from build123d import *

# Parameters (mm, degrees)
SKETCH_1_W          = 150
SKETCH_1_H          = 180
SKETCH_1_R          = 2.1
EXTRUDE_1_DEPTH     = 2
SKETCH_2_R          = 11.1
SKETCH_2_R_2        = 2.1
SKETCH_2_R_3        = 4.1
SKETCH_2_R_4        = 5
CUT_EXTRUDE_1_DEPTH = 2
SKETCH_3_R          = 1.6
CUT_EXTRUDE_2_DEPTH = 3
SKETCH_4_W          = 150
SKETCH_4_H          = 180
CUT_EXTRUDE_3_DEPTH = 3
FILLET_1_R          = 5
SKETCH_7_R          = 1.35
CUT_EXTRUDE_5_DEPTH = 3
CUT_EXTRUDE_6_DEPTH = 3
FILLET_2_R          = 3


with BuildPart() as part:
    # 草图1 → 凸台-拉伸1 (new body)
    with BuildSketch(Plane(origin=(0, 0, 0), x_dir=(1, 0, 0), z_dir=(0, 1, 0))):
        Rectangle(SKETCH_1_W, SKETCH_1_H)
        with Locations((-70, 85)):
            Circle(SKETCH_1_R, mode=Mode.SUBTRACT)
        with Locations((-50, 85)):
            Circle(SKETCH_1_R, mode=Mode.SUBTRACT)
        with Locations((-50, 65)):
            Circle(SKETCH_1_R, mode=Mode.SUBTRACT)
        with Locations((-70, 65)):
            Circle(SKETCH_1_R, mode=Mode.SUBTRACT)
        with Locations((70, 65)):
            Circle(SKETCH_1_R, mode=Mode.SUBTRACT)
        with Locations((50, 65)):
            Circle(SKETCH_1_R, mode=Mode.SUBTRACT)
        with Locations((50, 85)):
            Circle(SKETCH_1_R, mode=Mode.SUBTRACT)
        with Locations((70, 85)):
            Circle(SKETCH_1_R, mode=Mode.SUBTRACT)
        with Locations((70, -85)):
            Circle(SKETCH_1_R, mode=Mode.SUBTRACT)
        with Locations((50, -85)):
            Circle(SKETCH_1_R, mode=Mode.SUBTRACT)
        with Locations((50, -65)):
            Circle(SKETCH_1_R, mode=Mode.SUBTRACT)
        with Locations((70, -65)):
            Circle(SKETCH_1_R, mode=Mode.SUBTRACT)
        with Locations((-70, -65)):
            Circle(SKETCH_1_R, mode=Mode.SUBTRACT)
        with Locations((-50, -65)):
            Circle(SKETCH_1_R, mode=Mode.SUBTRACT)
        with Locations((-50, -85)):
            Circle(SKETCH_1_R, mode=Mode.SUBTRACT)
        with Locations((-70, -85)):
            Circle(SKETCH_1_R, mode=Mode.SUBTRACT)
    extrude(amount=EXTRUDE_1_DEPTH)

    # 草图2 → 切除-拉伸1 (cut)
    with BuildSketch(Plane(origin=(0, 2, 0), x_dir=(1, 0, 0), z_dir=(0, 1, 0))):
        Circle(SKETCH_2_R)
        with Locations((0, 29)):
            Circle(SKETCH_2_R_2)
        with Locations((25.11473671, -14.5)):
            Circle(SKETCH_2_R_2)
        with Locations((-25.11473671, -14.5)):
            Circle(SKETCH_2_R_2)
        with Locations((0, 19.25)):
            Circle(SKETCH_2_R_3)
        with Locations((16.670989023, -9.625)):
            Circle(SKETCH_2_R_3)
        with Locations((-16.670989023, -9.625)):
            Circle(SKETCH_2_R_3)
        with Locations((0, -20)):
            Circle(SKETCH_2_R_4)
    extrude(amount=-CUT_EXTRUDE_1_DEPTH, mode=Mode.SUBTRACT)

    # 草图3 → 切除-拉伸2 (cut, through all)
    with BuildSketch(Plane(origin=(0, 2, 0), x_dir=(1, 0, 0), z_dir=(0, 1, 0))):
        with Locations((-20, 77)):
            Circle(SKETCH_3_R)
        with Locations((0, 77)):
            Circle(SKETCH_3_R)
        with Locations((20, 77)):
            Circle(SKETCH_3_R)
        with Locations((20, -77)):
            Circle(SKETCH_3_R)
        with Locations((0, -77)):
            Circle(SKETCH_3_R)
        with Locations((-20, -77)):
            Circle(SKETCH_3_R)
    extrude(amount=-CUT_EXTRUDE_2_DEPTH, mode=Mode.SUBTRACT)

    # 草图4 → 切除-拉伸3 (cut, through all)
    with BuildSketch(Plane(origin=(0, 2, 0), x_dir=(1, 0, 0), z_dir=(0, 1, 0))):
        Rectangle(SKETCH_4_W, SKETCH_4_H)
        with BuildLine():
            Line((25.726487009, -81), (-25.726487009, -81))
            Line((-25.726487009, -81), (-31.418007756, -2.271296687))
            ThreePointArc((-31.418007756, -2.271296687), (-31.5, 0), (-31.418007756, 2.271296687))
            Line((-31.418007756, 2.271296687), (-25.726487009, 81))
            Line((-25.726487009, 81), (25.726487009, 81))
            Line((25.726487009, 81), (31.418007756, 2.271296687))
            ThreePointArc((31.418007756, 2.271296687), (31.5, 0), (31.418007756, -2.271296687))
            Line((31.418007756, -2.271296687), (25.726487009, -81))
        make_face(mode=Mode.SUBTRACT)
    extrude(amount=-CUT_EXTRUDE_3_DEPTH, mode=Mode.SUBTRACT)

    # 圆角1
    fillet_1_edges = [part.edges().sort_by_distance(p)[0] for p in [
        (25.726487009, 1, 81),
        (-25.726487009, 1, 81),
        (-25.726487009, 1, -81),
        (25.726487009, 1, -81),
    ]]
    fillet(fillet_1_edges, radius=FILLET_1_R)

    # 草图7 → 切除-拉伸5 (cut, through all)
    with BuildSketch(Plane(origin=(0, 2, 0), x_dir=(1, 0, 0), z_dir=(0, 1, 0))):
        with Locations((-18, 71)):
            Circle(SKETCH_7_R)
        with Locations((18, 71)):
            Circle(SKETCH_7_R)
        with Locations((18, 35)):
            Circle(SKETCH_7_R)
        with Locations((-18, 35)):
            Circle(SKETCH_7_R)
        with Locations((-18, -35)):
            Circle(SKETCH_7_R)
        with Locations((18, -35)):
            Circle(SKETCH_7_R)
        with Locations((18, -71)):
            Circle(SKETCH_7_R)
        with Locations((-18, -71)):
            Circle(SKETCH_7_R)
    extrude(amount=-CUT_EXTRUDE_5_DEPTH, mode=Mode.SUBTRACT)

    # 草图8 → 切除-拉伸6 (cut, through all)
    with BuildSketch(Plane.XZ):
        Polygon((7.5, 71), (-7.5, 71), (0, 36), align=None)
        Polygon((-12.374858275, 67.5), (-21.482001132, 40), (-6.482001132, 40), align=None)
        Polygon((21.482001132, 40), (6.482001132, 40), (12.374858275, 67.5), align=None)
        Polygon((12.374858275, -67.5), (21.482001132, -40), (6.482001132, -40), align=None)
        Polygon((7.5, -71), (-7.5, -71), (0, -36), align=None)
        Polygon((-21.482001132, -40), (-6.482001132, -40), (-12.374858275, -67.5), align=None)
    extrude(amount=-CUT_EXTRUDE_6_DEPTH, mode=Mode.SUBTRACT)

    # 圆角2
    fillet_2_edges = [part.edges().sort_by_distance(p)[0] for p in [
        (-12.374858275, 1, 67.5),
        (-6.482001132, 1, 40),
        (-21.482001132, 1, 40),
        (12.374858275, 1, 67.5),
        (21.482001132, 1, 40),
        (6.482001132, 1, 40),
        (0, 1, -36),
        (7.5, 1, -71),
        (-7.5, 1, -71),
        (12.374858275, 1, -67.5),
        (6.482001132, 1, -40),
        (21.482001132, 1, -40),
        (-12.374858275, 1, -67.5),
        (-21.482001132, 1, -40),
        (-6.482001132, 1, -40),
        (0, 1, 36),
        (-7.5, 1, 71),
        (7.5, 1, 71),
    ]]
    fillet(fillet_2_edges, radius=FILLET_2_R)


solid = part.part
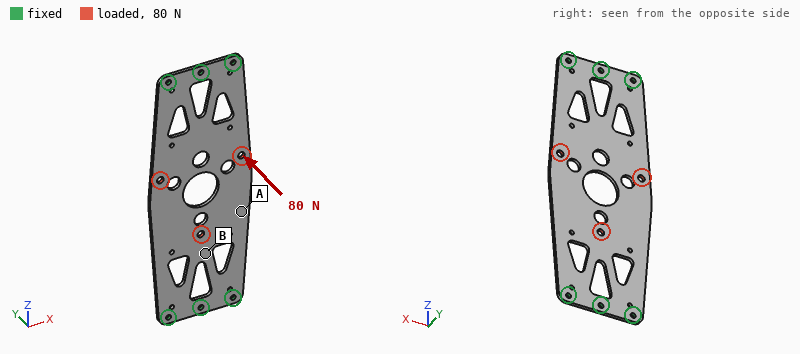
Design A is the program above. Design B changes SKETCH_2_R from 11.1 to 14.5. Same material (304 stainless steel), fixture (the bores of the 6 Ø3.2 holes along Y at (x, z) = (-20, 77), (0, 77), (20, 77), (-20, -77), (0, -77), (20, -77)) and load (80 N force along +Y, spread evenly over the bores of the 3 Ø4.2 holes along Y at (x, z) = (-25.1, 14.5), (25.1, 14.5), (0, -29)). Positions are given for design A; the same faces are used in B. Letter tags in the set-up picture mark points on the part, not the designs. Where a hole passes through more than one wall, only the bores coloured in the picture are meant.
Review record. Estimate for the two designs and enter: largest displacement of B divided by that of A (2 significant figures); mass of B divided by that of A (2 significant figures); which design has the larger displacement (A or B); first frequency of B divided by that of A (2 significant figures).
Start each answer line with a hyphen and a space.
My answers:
- 1.1
- 0.96
- B
- 1.0
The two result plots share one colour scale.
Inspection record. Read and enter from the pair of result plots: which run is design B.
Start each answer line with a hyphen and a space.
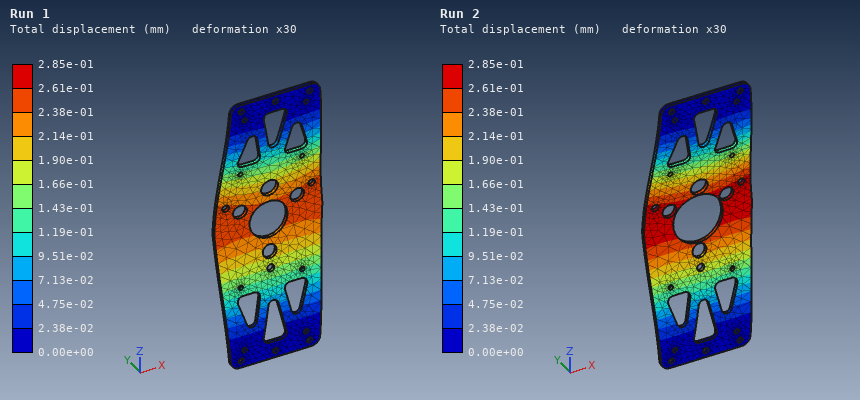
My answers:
- Run 2
